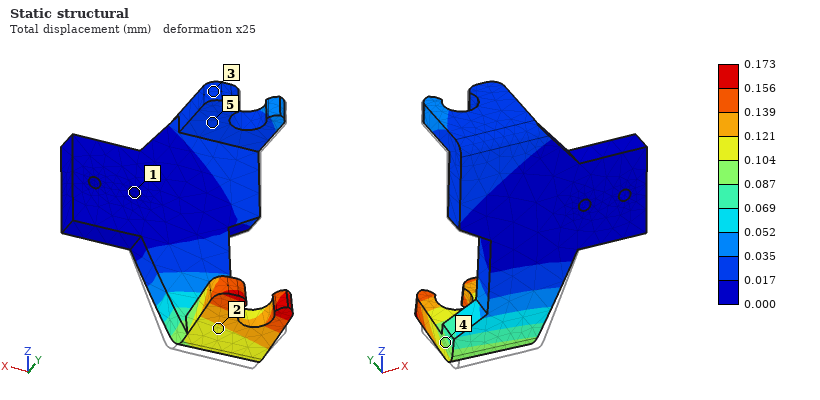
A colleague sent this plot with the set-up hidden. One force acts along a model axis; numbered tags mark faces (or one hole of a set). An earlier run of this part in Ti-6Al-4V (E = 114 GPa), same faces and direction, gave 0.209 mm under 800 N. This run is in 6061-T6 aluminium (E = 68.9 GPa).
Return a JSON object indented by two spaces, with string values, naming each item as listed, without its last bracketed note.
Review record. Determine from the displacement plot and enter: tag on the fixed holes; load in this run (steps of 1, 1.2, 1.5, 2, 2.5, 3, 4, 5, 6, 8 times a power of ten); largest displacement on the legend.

{
  "tag on the fixed holes": "1",
  "load in this run": "400 N",
  "largest displacement on the legend": "0.173 mm"
}
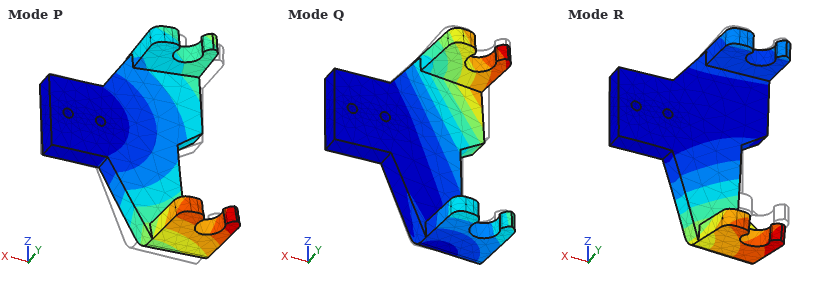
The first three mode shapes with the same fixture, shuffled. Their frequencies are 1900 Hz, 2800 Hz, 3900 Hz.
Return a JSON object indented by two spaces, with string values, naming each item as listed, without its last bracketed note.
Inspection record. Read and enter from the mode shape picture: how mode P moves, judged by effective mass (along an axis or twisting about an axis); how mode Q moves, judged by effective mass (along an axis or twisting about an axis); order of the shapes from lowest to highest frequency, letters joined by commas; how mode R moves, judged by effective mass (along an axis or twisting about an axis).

{
  "how mode P moves, judged by effective mass": "along Z",
  "how mode Q moves, judged by effective mass": "along Y",
  "order of the shapes from lowest to highest frequency, letters joined by commas": "R, Q, P",
  "how mode R moves, judged by effective mass": "along Y"
}
